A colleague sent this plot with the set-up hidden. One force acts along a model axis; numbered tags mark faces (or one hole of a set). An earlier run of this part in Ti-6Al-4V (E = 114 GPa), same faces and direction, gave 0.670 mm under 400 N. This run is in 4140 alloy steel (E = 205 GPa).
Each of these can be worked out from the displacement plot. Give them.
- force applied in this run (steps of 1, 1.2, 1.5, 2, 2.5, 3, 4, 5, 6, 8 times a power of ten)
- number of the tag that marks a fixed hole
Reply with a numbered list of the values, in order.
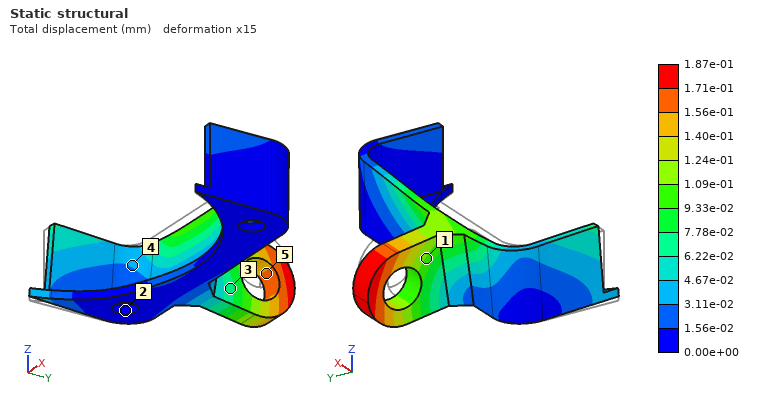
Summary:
1. 200 N
2. 2
